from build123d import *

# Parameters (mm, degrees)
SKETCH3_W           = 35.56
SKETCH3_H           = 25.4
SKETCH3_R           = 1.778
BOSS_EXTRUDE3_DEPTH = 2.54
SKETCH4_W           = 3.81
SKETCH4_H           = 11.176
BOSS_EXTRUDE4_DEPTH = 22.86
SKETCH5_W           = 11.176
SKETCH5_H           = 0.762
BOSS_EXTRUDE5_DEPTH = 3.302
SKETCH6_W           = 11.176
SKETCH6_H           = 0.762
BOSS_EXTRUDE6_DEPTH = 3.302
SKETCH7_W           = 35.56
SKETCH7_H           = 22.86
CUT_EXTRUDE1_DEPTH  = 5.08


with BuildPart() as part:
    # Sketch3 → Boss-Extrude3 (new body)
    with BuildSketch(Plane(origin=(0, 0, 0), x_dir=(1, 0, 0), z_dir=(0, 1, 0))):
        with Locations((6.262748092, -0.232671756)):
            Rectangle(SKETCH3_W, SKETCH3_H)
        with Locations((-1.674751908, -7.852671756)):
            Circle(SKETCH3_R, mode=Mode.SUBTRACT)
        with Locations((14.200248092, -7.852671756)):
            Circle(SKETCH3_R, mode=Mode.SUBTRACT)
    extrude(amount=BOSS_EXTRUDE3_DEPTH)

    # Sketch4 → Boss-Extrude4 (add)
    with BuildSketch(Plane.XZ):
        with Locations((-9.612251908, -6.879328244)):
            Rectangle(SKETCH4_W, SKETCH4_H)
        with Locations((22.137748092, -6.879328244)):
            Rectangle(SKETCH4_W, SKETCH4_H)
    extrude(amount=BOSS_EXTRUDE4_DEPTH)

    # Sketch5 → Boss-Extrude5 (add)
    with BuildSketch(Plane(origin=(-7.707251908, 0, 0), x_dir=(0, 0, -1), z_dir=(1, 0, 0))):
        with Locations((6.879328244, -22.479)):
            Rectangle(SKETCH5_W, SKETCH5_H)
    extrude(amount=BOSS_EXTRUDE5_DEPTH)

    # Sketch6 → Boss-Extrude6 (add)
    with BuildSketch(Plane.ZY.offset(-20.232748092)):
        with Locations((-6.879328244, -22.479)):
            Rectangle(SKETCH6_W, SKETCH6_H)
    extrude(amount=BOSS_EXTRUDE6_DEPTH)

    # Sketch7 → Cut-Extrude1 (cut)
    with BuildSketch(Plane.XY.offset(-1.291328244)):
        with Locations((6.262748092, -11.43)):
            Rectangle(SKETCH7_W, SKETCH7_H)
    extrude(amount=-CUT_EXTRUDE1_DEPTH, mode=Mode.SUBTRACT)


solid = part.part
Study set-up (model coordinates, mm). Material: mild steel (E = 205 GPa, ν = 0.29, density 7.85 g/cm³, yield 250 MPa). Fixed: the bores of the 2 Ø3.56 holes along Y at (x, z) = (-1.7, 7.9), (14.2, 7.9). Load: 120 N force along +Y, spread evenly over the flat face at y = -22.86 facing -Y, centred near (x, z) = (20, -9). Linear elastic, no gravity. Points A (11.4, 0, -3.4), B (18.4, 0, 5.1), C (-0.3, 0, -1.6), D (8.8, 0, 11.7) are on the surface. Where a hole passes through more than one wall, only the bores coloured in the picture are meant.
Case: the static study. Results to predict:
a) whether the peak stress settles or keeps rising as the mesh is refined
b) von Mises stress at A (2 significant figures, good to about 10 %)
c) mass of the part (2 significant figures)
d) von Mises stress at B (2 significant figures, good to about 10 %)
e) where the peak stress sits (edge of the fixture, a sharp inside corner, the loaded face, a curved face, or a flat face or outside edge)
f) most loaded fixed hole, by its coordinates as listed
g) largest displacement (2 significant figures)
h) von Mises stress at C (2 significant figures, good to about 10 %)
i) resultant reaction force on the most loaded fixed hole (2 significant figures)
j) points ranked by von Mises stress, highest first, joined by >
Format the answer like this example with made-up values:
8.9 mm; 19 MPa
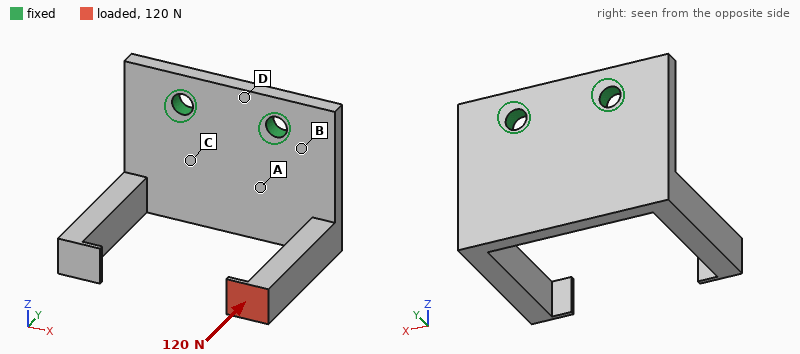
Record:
keeps rising; 41 MPa; 26 g; 65 MPa; edge of the fixture; (14.2, 7.9); 91 µm; 23 MPa; 140 N; B > A > C > D
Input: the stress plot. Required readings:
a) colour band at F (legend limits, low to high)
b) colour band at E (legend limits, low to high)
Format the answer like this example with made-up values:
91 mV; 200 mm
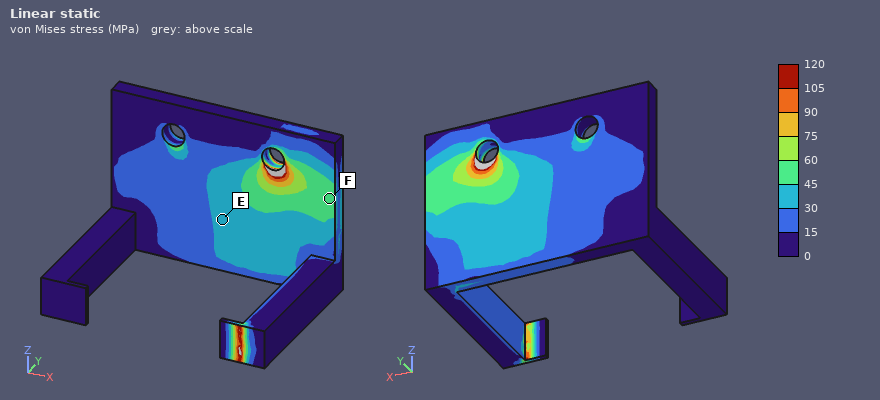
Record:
45 to 60 MPa; 30 to 45 MPa
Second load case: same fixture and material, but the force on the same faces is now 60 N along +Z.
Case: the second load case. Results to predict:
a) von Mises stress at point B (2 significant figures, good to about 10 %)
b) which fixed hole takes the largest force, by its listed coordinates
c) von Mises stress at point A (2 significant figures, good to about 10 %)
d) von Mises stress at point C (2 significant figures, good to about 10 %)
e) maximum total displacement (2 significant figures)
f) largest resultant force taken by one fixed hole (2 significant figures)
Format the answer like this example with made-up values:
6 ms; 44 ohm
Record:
47 MPa; (14.2, 7.9); 48 MPa; 24 MPa; 0.14 mm; 76 N
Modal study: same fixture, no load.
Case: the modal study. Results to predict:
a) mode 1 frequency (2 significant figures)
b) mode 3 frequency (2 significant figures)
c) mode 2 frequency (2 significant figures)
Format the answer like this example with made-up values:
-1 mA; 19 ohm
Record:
2100 Hz; 2700 Hz; 2200 Hz
